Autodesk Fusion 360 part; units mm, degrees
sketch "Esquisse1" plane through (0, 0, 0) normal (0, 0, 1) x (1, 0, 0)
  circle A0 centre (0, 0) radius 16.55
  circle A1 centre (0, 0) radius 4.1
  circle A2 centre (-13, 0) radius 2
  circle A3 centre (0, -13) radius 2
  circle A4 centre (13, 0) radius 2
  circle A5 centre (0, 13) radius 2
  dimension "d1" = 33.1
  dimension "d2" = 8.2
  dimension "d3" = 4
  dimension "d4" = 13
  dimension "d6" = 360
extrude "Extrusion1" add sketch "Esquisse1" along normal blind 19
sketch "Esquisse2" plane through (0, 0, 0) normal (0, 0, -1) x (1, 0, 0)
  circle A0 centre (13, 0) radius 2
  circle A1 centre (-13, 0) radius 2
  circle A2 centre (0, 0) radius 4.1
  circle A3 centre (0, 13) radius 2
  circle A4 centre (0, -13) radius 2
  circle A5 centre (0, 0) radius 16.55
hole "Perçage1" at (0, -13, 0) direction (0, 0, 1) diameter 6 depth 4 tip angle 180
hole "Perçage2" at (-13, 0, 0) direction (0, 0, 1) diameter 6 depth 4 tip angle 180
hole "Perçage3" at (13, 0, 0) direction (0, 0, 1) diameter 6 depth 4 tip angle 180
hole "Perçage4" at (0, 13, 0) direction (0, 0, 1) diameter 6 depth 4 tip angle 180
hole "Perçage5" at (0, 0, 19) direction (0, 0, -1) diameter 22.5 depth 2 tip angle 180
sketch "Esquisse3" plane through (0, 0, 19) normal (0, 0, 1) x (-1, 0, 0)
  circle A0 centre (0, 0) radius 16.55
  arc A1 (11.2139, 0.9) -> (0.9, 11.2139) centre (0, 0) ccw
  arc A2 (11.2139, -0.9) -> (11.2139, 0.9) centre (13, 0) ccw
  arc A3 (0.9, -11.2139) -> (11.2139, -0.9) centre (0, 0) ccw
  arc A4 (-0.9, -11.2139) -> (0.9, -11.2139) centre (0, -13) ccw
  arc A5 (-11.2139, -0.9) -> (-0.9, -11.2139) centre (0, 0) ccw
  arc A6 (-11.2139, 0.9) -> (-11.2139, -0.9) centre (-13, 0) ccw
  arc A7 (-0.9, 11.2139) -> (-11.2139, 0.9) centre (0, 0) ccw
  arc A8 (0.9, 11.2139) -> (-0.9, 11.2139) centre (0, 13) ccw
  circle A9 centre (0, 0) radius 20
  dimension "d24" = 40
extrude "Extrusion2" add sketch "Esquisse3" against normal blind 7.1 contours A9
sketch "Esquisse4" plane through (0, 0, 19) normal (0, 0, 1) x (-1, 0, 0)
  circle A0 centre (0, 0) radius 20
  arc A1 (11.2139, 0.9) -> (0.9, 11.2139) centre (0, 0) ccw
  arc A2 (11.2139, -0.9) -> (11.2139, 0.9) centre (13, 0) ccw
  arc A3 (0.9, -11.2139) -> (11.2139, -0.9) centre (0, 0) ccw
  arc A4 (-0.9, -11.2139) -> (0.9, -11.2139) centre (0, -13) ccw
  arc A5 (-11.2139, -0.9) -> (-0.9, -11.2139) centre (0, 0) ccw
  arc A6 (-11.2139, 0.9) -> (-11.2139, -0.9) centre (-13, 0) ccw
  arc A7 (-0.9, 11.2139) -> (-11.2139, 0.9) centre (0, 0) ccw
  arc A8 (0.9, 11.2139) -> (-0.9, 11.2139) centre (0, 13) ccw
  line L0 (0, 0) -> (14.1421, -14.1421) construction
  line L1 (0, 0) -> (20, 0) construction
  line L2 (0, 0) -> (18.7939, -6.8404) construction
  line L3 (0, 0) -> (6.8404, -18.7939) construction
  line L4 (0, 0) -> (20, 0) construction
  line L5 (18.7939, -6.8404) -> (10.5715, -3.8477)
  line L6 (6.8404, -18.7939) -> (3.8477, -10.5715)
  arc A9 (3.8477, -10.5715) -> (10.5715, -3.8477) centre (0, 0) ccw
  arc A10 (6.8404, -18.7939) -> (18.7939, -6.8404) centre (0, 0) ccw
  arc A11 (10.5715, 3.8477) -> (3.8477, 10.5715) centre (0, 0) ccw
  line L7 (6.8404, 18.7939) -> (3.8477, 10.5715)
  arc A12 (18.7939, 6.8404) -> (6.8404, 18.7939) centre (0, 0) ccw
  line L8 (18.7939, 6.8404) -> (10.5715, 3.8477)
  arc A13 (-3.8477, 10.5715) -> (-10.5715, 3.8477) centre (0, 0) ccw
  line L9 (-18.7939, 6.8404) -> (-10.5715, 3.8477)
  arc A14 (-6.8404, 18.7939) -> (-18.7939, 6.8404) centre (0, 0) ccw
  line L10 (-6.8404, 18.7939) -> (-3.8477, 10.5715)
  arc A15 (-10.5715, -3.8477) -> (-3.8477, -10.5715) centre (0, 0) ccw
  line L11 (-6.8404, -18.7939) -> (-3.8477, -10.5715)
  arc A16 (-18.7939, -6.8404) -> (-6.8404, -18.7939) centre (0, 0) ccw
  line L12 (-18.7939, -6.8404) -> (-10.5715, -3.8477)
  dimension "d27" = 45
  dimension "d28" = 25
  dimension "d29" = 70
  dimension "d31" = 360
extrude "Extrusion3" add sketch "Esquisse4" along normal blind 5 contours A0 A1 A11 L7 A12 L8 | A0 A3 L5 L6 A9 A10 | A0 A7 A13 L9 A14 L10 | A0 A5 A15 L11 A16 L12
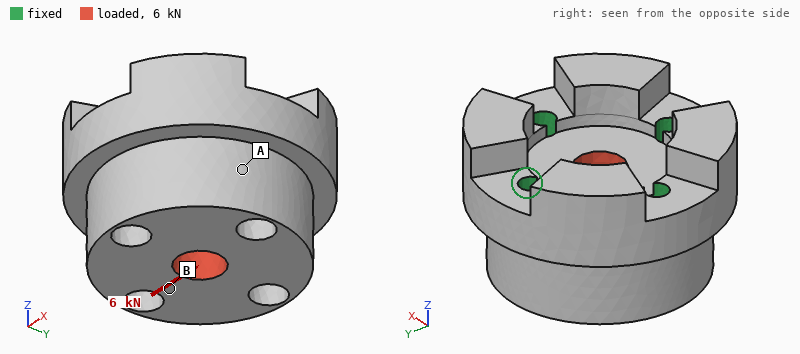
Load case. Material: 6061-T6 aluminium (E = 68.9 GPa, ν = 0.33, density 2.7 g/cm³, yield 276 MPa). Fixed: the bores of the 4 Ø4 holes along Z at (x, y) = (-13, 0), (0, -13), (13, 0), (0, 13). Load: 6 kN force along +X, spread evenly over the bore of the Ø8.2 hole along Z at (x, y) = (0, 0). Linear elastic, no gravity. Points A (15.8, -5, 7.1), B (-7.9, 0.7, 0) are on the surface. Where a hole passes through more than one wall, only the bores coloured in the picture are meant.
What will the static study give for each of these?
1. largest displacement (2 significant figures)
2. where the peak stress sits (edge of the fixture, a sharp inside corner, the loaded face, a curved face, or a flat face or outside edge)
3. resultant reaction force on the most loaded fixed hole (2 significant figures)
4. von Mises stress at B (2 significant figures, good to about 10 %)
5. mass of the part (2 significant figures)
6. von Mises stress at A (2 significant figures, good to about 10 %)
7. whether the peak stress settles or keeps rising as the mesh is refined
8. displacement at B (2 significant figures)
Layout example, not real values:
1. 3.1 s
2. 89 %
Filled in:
1. 3.0 µm
2. edge of the fixture
3. 1.9 kN
4. 11 MPa
5. 50 g
6. 4.7 MPa
7. keeps rising
8. 2.3 µm
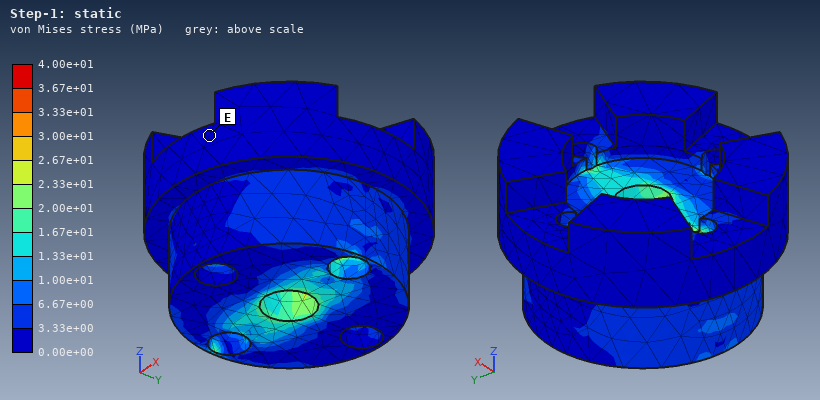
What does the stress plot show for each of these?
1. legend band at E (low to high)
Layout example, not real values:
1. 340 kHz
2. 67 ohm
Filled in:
1. 0.00e+00 to 3.33e+00 MPa
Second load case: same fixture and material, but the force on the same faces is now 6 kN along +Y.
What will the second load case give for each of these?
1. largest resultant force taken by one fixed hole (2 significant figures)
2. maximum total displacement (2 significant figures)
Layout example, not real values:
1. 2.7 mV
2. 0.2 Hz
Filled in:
1. 1.9 kN
2. 3.0 µm
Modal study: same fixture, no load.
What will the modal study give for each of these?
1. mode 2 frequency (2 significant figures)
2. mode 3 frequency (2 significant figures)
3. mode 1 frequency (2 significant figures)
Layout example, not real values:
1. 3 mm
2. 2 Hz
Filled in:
1. 38 kHz
2. 38 kHz
3. 37 kHz
